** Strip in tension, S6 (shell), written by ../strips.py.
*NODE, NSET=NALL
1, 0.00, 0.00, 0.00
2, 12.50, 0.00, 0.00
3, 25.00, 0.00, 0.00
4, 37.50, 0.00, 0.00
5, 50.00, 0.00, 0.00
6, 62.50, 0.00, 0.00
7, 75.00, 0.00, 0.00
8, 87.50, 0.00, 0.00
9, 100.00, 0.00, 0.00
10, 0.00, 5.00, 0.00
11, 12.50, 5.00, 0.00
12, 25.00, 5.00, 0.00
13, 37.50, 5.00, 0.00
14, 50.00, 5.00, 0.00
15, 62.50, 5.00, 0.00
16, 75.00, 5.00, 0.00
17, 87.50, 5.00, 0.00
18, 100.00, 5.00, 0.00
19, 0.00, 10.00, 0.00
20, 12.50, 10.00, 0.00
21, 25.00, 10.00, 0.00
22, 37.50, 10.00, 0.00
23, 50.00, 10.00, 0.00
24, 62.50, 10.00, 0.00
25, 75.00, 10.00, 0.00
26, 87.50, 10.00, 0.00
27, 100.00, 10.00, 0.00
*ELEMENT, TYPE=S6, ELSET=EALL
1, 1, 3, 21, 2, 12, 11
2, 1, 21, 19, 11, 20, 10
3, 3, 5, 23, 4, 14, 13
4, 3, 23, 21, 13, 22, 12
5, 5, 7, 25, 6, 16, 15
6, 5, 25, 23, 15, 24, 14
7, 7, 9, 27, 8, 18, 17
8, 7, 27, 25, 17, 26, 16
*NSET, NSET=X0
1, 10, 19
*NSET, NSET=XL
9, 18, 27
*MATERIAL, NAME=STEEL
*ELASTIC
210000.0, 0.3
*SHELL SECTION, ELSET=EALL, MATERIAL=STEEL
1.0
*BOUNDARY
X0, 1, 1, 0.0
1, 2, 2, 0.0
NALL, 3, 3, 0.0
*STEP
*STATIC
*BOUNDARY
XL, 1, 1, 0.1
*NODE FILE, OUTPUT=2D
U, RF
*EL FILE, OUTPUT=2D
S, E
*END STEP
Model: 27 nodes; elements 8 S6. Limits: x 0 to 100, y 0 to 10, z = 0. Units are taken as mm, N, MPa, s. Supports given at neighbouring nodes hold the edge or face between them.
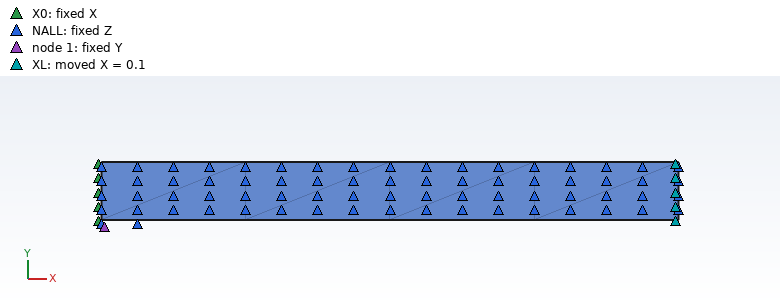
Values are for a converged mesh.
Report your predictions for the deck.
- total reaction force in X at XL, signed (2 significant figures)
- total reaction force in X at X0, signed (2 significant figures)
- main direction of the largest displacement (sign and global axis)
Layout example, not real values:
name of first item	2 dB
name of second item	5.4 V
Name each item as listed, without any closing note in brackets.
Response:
total reaction force in X at XL, signed	2100 N
total reaction force in X at X0, signed	-2100 N
main direction of the largest displacement	+X
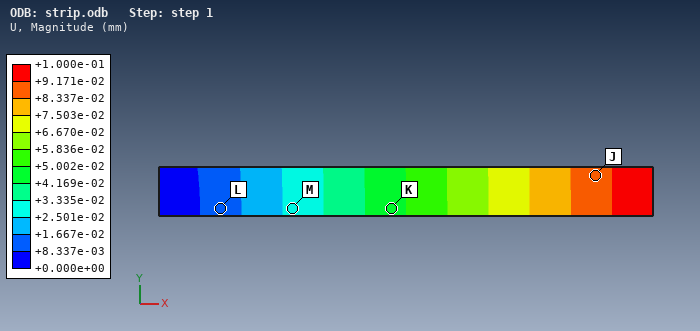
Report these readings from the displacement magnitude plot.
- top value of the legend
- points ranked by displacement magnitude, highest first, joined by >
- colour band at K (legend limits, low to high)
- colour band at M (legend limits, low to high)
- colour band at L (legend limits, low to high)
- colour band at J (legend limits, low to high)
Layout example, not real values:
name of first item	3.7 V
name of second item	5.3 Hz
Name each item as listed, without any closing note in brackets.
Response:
top value of the legend	+1.000e-01 mm
points ranked by displacement magnitude, highest first, joined by >	J > K > M > L
colour band at K	+4.169e-02 to +5.002e-02 mm
colour band at M	+2.501e-02 to +3.335e-02 mm
colour band at L	+8.337e-03 to +1.667e-02 mm
colour band at J	+8.337e-02 to +9.171e-02 mm
